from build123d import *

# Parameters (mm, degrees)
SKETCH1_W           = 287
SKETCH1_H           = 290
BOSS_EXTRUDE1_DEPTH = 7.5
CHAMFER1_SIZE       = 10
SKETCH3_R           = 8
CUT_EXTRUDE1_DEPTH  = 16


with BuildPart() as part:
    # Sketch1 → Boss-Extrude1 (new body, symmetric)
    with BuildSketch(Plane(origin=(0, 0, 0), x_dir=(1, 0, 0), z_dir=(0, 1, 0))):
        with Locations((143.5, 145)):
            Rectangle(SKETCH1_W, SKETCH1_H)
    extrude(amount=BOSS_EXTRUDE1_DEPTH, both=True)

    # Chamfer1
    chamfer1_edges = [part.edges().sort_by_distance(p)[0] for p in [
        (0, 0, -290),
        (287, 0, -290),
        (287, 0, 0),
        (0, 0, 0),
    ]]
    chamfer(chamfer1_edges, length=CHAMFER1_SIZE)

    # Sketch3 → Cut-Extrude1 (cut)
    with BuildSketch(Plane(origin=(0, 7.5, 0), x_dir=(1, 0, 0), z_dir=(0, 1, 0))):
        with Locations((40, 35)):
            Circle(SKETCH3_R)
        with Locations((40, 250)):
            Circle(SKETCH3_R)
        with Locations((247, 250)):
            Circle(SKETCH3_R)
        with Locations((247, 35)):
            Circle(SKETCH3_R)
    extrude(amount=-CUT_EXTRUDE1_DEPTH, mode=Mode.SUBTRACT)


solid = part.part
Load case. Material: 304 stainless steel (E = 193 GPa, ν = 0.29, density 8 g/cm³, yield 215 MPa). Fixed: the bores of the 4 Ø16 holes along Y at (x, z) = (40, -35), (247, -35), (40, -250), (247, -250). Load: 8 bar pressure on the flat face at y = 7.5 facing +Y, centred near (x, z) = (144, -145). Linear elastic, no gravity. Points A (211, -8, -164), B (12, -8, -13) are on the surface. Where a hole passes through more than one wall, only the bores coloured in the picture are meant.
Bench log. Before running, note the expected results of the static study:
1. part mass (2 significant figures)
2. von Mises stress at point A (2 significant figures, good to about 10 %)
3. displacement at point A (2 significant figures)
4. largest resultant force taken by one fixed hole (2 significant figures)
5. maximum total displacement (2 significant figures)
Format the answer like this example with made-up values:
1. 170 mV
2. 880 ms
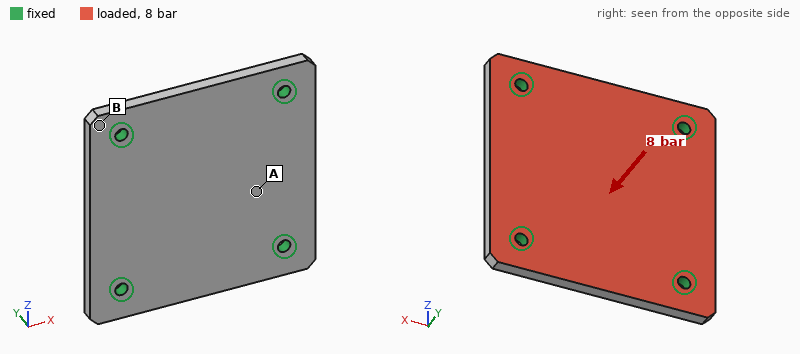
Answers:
1. 9.9 kg
2. 40 MPa
3. 0.14 mm
4. 17 kN
5. 0.19 mm
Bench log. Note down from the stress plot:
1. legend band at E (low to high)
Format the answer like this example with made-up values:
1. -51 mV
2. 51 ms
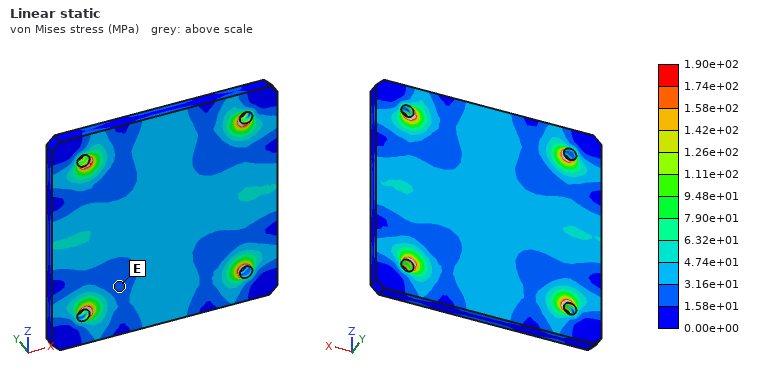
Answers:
1. 1.58e+01 to 3.16e+01 MPa
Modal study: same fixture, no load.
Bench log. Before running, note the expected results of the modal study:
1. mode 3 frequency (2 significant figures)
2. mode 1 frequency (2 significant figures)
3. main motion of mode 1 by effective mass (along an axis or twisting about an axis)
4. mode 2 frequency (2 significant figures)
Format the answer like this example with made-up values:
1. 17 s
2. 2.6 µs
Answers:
1. 1800 Hz
2. 1200 Hz
3. along Y
4. 1700 Hz
